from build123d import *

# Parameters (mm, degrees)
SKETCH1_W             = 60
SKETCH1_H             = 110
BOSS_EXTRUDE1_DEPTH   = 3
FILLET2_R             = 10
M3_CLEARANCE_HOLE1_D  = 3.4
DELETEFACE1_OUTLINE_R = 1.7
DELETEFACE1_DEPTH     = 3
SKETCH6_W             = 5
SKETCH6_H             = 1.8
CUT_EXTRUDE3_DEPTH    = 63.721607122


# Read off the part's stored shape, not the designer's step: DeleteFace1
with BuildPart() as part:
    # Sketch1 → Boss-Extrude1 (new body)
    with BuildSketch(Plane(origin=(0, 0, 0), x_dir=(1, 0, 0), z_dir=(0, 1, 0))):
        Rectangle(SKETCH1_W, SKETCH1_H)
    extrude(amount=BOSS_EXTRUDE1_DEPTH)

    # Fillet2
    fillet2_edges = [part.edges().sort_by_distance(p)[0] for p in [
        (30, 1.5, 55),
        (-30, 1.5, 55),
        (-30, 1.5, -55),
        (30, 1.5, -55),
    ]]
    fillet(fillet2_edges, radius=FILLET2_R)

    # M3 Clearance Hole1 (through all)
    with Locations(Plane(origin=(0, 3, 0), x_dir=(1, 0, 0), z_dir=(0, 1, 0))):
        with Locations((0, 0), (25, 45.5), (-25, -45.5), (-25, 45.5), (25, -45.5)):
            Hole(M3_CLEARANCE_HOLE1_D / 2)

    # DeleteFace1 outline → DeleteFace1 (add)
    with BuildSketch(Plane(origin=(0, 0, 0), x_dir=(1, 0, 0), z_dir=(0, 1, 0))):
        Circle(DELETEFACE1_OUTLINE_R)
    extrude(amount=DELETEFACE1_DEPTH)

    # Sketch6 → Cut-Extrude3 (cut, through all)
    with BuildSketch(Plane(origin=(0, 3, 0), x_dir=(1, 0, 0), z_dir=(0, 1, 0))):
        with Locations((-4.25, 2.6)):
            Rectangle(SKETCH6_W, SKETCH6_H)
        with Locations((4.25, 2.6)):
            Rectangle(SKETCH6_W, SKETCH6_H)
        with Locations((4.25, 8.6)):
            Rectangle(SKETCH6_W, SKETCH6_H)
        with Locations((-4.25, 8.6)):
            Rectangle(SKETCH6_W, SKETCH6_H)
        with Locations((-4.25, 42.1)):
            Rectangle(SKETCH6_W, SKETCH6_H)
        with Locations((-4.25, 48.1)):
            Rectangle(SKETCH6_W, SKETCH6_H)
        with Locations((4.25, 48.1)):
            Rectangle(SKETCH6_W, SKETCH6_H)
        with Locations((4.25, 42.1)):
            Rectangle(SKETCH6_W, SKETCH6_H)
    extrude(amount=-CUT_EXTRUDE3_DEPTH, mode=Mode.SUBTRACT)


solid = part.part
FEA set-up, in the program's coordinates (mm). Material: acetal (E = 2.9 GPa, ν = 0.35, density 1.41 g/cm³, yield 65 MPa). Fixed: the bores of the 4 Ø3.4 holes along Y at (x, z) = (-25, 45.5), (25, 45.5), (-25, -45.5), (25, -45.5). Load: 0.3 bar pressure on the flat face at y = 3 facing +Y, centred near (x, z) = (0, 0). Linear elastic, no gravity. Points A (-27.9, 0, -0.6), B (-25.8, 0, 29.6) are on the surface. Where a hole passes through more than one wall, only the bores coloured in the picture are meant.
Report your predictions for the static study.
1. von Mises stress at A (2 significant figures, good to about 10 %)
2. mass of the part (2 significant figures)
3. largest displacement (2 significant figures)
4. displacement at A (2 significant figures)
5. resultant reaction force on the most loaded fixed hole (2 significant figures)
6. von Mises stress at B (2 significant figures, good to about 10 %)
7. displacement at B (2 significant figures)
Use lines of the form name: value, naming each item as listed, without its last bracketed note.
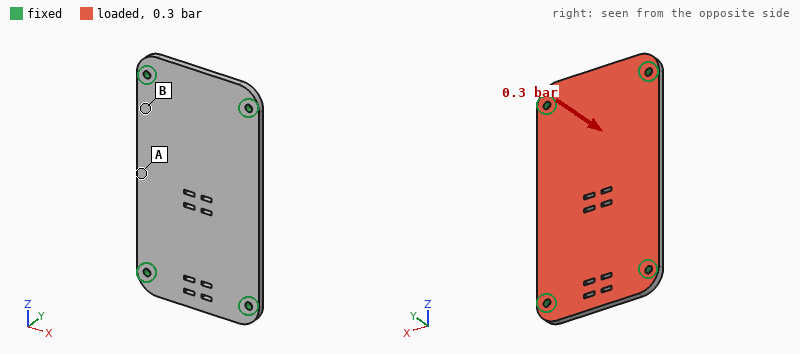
von Mises stress at A: 8.9 MPa
mass of the part: 27 g
largest displacement: 1.1 mm
displacement at A: 1.1 mm
resultant reaction force on the most loaded fixed hole: 48 N
von Mises stress at B: 2.7 MPa
displacement at B: 0.38 mm
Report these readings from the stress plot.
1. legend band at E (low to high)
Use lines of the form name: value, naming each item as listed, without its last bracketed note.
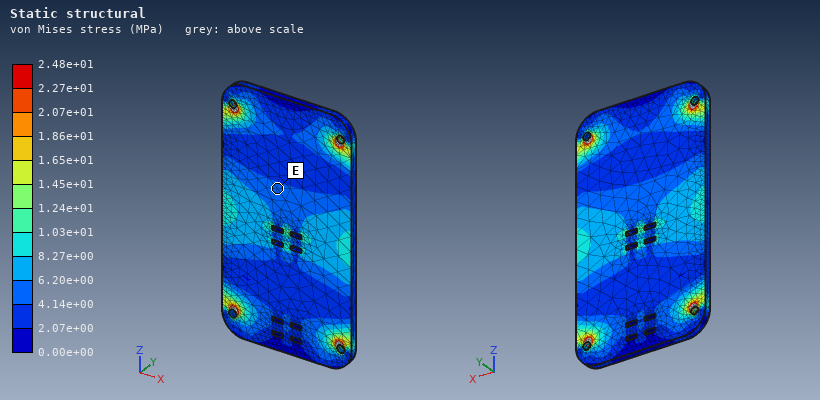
legend band at E: 4.14e+00 to 6.20e+00 MPa
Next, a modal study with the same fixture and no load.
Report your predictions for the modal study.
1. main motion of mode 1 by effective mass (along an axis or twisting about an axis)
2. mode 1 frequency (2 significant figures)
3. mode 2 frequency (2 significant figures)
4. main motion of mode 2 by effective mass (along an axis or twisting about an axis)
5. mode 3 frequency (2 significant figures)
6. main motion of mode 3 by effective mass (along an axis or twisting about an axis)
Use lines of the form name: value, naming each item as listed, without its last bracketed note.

main motion of mode 1 by effective mass: along Y
mode 1 frequency: 460 Hz
mode 2 frequency: 750 Hz
main motion of mode 2 by effective mass: twisting about Z
mode 3 frequency: 1200 Hz
main motion of mode 3 by effective mass: twisting about X
